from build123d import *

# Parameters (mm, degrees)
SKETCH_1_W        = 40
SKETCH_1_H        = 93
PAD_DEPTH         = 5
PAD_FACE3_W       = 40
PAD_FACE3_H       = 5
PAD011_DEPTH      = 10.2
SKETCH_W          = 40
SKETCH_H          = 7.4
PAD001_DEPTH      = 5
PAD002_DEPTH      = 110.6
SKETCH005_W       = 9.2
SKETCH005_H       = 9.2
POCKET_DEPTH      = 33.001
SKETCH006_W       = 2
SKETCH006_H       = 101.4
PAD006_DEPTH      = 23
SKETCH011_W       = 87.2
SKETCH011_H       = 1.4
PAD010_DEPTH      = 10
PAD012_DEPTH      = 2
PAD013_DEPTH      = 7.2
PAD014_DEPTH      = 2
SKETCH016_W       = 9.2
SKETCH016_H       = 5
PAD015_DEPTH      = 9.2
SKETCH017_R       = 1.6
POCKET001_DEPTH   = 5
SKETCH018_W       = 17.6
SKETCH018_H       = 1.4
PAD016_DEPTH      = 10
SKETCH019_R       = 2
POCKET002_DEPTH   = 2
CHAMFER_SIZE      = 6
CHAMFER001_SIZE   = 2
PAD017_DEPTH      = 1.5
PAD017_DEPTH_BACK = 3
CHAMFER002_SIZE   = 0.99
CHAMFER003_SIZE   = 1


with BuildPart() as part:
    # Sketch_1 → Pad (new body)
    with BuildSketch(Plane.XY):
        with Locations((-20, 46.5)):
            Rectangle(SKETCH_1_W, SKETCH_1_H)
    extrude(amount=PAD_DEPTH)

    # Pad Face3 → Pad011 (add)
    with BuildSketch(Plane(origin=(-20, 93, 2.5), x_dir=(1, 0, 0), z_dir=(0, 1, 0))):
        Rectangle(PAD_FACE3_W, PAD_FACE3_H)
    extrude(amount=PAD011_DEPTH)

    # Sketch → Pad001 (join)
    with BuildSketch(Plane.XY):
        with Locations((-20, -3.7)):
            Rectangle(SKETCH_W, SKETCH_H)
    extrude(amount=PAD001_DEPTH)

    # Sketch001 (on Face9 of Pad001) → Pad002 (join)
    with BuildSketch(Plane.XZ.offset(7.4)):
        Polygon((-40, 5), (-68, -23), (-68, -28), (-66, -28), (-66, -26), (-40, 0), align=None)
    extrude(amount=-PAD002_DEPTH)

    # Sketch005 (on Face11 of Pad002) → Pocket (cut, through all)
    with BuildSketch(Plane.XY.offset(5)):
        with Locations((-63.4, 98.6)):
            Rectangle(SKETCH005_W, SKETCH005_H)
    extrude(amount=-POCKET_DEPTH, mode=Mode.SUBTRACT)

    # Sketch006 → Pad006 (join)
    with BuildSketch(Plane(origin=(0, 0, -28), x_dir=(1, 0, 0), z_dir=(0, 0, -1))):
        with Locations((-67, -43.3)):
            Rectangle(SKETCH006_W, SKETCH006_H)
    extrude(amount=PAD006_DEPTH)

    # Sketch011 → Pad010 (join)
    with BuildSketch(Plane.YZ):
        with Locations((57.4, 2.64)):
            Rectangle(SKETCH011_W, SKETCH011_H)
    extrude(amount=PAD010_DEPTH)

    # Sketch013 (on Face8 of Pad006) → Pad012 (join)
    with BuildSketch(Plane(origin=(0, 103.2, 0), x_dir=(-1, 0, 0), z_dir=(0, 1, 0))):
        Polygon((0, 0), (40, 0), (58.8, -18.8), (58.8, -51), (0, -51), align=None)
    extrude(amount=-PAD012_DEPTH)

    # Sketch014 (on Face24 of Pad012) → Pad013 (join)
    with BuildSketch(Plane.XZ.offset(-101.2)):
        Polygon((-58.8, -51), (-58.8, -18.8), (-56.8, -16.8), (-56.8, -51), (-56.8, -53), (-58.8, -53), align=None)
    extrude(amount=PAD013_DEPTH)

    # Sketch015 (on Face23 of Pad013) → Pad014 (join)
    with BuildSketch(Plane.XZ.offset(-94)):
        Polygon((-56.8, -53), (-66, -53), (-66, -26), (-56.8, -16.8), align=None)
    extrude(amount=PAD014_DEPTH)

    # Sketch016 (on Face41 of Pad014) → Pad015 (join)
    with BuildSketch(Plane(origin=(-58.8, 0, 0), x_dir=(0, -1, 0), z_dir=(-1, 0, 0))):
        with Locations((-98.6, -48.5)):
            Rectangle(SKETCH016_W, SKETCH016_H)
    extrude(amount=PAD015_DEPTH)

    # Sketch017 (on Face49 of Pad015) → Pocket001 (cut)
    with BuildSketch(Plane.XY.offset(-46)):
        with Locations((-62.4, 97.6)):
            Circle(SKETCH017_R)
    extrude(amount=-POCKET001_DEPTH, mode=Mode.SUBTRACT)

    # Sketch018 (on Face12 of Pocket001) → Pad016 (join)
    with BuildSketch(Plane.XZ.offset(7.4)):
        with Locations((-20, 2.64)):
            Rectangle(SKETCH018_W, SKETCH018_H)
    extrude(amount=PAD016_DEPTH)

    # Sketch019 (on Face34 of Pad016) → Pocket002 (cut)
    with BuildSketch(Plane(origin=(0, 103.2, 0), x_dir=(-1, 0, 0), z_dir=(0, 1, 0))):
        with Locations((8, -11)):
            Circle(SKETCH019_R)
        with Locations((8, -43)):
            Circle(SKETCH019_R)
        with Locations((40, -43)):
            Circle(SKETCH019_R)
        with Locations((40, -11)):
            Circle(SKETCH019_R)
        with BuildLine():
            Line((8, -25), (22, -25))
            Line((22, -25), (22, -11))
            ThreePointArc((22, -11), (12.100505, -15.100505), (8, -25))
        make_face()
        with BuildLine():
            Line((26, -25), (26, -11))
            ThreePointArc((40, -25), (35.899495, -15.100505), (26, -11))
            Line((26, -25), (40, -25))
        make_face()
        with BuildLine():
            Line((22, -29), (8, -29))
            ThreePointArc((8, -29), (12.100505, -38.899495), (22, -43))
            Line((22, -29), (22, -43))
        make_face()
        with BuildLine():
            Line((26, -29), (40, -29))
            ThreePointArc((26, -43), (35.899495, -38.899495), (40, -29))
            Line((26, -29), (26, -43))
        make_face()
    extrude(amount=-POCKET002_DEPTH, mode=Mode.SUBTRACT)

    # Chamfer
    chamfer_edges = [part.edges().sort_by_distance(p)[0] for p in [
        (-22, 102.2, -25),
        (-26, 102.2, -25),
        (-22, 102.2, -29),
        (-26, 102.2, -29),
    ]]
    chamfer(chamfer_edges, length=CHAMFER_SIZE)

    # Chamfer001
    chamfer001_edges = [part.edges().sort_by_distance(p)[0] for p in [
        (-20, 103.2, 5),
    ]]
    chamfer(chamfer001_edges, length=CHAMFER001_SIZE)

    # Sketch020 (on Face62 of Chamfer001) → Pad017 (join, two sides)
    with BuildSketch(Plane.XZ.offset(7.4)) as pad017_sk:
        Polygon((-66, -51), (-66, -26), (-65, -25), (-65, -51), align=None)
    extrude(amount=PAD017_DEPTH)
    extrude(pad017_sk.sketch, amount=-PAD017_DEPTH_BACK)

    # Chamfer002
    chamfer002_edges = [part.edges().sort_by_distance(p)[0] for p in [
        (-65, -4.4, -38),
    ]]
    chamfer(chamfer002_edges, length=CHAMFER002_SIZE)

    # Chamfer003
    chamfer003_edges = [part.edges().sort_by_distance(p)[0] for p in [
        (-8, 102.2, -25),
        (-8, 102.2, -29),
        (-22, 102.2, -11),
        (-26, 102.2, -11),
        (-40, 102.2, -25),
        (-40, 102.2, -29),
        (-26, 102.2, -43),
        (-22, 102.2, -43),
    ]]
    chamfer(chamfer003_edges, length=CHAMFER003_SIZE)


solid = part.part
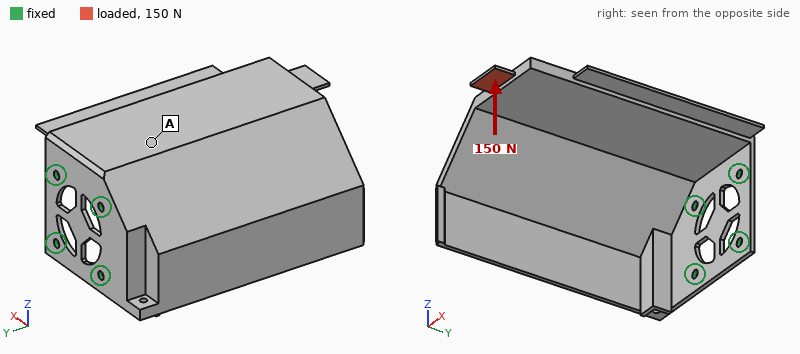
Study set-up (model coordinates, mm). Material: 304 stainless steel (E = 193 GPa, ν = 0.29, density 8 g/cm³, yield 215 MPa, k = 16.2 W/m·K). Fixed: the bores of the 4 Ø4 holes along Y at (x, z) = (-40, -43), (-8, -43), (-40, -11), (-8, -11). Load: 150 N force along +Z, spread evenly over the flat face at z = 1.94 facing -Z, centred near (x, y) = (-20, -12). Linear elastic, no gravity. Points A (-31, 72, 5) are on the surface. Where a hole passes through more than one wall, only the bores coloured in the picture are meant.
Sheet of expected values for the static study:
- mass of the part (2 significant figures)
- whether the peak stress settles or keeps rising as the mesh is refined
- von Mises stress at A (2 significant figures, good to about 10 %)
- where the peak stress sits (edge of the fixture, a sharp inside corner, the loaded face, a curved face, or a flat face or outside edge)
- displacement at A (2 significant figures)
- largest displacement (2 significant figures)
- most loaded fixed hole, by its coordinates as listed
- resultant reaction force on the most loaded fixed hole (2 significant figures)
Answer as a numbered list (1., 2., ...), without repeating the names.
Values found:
1. 400 g
2. keeps rising
3. 25 MPa
4. edge of the fixture
5. 0.20 mm
6. 0.84 mm
7. (-40, -11)
8. 500 N
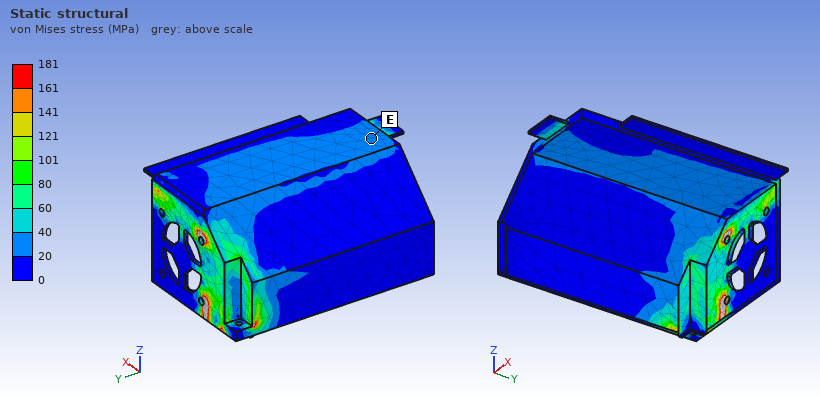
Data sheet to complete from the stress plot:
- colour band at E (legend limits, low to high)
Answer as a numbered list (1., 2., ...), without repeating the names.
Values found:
1. 20 to 40 MPa
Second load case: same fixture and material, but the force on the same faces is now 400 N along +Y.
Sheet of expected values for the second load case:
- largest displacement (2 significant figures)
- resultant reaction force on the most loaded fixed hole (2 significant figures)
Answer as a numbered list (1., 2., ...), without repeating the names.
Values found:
1. 0.13 mm
2. 240 N
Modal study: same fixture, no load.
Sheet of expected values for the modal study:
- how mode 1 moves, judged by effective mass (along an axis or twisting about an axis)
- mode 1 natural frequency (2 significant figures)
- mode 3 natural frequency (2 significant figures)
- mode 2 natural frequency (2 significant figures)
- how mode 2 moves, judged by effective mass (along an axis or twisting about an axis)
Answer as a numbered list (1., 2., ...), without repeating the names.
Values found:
1. along Z
2. 230 Hz
3. 820 Hz
4. 400 Hz
5. along X
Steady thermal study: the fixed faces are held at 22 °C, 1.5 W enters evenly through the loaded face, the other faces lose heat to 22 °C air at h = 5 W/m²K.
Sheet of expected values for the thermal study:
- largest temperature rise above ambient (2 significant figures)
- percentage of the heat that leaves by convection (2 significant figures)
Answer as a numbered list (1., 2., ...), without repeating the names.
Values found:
1. 45 K
2. 72 %
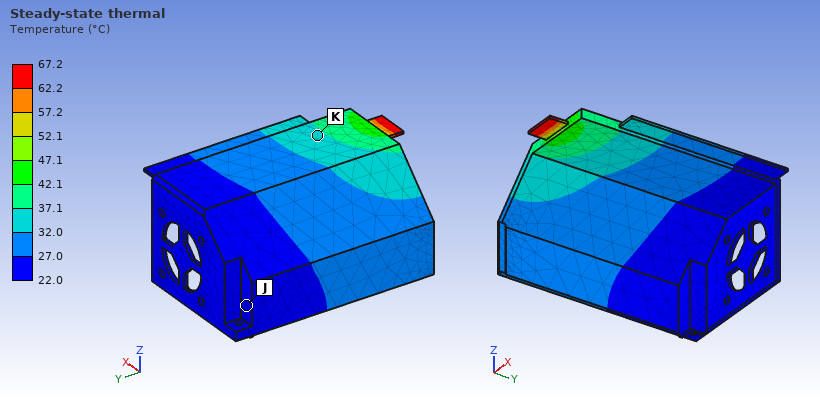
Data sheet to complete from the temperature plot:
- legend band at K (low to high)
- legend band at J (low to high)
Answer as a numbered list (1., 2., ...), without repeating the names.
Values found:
1. 32.0 to 37.1 °C
2. 22.0 to 27.0 °C
